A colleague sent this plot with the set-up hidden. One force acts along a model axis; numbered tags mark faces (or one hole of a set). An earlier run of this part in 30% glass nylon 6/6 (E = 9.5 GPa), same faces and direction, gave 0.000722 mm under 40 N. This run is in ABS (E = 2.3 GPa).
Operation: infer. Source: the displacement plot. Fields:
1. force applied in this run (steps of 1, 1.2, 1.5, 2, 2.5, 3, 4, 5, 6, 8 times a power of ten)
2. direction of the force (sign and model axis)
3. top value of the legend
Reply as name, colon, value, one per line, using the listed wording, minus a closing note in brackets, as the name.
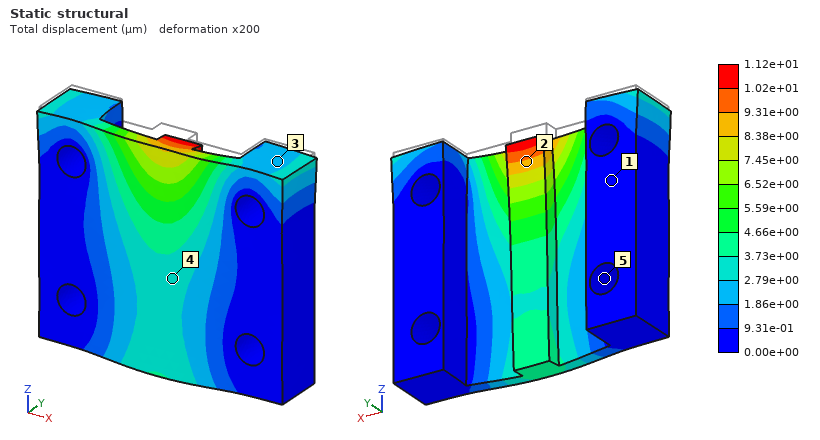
force applied in this run: 150 N
direction of the force: -Z
top value of the legend: 1.12e+01 µm
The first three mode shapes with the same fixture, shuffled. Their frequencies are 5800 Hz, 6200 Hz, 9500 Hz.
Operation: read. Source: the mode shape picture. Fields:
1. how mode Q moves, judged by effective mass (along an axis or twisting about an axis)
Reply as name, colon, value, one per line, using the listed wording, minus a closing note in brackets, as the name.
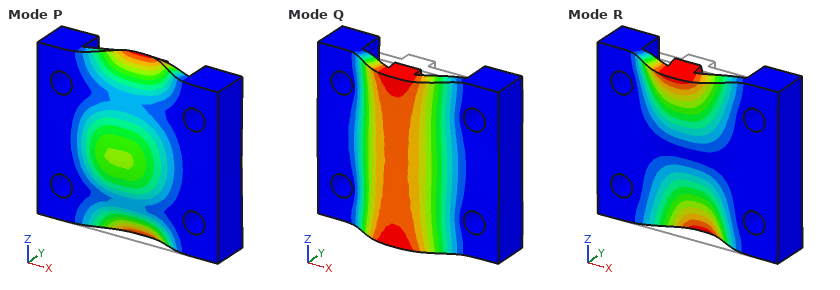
how mode Q moves, judged by effective mass: along Y
